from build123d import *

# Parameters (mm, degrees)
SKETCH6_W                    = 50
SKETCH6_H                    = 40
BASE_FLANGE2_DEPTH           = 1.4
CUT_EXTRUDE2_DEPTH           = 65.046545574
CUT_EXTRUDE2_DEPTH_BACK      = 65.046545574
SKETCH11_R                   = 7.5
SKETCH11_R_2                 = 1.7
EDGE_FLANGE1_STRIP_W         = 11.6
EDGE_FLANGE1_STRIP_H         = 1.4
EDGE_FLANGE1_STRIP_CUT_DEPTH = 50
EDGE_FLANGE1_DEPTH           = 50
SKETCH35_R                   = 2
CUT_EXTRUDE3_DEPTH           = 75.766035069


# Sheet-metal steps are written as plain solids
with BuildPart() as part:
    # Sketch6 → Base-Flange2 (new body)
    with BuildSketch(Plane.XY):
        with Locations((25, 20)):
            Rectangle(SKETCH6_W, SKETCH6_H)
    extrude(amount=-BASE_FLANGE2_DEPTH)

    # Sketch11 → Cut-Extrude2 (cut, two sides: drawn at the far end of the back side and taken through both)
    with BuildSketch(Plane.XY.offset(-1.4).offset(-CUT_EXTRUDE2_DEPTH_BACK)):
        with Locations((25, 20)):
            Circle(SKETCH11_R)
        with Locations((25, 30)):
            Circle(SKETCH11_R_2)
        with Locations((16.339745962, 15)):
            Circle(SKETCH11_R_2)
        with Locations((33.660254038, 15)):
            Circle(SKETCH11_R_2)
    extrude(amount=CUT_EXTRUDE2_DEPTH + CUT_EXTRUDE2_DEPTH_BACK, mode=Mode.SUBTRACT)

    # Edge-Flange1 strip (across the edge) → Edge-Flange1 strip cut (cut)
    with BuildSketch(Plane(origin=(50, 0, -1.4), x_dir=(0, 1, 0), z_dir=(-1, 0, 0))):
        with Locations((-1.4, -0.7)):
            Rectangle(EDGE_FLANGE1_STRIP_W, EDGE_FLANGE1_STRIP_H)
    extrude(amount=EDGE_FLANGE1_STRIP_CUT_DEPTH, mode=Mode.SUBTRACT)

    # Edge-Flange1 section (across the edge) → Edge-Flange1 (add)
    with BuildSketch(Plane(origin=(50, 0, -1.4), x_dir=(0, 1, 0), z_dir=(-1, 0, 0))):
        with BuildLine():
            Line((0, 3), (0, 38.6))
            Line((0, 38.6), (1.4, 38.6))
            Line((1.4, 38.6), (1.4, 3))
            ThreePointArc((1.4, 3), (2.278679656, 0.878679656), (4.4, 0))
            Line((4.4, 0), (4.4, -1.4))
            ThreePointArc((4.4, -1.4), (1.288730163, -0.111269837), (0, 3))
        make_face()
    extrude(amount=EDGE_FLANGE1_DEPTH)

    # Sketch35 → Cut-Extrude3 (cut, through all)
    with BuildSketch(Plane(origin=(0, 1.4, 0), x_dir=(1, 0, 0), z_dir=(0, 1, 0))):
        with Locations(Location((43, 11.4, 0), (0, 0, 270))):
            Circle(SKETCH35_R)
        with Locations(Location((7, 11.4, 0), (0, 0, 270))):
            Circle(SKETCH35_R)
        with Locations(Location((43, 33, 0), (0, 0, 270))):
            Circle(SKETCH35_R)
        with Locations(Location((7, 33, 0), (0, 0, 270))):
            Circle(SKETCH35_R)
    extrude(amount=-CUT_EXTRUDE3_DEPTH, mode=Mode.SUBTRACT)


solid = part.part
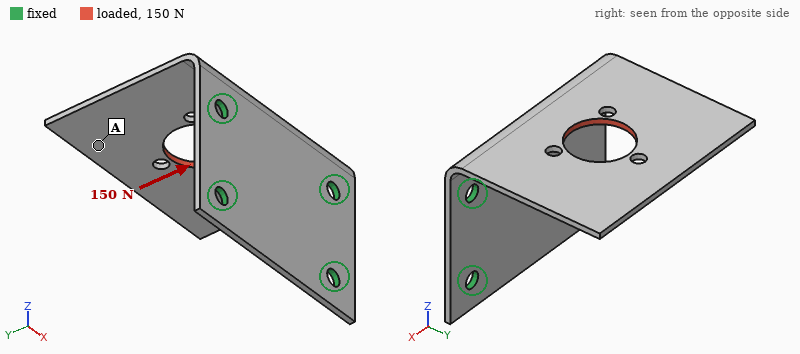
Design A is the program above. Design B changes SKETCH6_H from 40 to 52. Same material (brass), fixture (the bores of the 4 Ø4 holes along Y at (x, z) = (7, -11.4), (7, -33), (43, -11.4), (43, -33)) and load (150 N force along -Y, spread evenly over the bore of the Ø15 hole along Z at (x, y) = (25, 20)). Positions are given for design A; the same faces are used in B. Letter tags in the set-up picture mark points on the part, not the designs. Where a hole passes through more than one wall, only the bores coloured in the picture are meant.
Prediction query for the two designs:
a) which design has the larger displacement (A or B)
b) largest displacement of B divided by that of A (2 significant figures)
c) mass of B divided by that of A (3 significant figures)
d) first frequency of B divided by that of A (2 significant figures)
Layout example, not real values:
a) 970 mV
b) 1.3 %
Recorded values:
a) B
b) 1.1
c) 1.08
d) 0.76
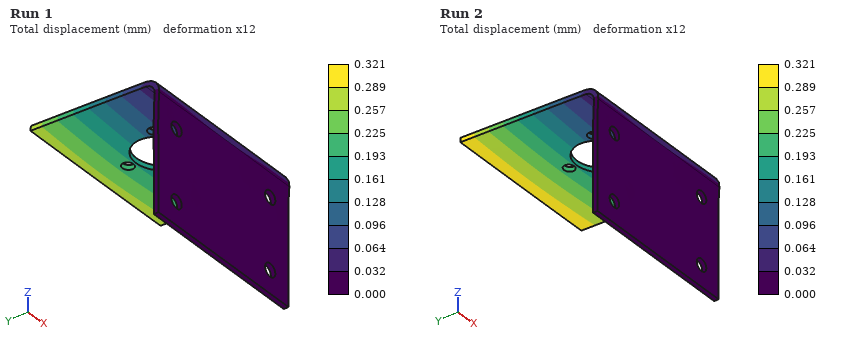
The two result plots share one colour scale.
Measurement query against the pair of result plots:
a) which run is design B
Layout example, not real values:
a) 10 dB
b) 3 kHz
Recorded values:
a) Run 2
